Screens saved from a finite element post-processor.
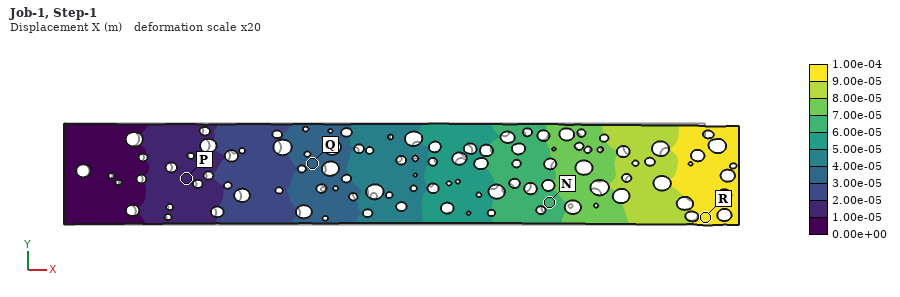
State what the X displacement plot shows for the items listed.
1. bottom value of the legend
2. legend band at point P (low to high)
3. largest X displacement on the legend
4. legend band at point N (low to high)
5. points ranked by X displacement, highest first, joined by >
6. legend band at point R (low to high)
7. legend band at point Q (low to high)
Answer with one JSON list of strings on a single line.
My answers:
["0.00e+00 m", "1.00e-05 to 2.00e-05 m", "1.00e-04 m", "6.00e-05 to 7.00e-05 m", "R > N > Q > P", "9.00e-05 to 1.00e-04 m", "3.00e-05 to 4.00e-05 m"]
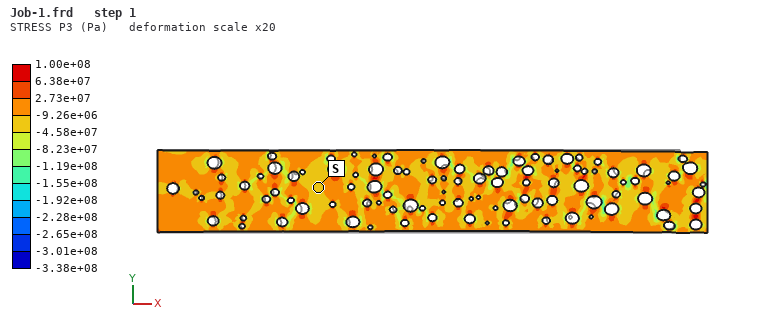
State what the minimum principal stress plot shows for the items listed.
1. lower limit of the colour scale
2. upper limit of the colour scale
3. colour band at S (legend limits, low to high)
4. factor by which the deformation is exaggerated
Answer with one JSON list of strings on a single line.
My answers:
["-3.38e+08 Pa", "1.00e+08 Pa", "-4.58e+07 to -9.26e+06 Pa", "20"]
